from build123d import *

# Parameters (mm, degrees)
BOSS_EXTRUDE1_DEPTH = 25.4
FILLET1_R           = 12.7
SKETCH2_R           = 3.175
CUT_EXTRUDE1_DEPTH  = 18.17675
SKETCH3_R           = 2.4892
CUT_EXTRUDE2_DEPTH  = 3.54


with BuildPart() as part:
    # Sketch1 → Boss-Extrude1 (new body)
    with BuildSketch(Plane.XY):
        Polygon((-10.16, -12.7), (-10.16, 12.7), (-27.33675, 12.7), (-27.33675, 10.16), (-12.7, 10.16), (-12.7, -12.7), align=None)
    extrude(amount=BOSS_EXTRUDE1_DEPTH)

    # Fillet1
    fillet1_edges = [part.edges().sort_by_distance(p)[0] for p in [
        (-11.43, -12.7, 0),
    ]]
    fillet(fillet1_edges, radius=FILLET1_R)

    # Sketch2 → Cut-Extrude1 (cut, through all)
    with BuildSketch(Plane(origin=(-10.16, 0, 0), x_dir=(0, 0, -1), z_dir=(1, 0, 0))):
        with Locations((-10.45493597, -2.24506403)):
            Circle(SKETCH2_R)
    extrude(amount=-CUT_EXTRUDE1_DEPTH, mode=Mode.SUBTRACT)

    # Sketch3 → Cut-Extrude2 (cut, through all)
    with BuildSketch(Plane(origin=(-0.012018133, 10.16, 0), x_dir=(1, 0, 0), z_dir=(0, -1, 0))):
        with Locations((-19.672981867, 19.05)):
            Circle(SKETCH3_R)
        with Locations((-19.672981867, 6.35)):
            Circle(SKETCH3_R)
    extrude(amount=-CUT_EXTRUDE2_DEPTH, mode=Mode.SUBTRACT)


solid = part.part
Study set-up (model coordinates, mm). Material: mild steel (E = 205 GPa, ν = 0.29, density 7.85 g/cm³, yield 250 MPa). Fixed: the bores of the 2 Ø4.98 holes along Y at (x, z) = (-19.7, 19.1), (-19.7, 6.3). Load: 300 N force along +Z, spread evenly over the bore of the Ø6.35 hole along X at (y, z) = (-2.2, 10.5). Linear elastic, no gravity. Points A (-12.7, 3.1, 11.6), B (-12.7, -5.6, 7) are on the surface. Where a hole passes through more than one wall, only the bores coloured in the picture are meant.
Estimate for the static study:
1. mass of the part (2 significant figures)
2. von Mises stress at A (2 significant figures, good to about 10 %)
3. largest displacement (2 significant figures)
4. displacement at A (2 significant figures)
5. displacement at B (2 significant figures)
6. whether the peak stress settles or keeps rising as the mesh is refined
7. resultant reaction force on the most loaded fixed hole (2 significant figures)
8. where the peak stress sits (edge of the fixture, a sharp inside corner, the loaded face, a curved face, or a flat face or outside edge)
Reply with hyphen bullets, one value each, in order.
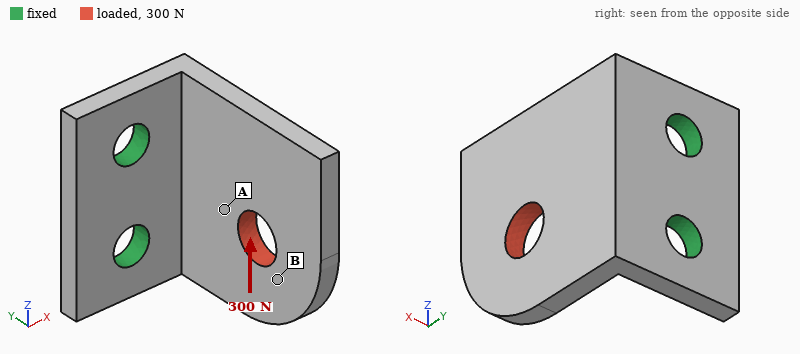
- 18 g
- 27 MPa
- 21 µm
- 6.8 µm
- 14 µm
- keeps rising
- 320 N
- edge of the fixture
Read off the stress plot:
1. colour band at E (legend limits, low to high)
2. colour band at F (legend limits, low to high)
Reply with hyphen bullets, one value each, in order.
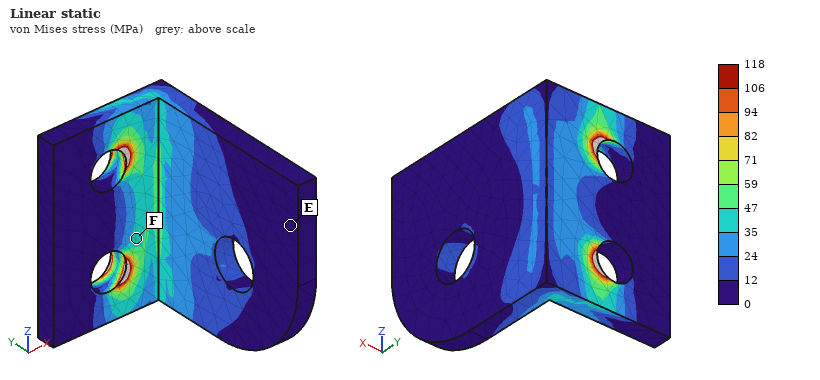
- 0 to 12 MPa
- 35 to 47 MPa
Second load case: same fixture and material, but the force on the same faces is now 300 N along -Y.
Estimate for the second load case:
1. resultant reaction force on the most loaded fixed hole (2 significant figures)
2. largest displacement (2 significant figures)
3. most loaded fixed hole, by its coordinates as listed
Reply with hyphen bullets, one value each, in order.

- 190 N
- 24 µm
- (-19.7, 6.3)
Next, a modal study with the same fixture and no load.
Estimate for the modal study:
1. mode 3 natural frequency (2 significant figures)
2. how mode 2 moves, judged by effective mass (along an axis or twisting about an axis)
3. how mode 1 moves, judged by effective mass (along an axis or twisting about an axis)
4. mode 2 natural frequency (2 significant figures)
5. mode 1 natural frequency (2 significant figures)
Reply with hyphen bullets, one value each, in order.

- 9700 Hz
- along Z
- along X
- 6900 Hz
- 2800 Hz
